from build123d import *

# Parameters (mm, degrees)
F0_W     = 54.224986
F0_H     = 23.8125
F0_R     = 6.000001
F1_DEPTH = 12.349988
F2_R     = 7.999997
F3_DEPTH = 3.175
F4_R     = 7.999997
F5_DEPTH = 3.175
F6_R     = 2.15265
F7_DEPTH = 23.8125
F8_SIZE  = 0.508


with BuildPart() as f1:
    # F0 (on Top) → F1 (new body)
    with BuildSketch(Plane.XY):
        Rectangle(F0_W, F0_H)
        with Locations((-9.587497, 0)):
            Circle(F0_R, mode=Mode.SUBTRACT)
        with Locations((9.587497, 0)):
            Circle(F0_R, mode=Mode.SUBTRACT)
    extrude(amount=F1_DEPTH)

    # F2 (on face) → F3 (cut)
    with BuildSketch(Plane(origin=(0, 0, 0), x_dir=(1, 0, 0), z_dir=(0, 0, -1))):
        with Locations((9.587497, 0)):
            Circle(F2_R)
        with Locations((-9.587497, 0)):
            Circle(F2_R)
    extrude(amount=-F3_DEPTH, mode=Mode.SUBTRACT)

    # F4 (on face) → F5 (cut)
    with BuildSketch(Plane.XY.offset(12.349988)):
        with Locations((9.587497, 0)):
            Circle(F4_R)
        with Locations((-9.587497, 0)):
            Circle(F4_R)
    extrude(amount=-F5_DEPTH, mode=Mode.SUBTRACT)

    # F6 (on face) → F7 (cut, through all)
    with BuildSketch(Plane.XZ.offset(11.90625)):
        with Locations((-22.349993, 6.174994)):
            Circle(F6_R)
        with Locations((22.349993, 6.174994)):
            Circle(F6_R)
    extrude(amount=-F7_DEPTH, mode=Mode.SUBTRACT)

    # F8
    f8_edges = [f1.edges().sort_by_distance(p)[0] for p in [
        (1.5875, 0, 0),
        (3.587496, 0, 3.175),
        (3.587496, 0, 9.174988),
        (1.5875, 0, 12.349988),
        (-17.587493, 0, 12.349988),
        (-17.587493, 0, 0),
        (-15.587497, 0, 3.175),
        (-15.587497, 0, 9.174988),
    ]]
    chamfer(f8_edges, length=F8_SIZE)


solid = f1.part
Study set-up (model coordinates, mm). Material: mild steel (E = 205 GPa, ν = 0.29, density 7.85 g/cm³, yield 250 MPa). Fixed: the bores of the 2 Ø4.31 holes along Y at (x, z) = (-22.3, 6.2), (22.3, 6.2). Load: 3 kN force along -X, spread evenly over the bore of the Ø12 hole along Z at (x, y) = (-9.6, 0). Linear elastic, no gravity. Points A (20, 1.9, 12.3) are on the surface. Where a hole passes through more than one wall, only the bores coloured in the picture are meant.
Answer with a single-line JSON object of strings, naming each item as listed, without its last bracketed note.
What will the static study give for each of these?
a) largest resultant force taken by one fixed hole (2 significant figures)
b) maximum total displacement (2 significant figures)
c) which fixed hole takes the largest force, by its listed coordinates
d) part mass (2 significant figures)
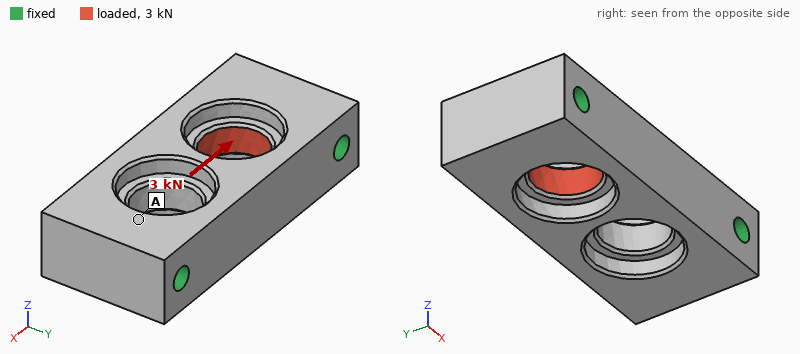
{"largest resultant force taken by one fixed hole": "2.2 kN", "maximum total displacement": "1.5 µm", "which fixed hole takes the largest force, by its listed coordinates": "(-22.3, 6.2)", "part mass": "89 g"}
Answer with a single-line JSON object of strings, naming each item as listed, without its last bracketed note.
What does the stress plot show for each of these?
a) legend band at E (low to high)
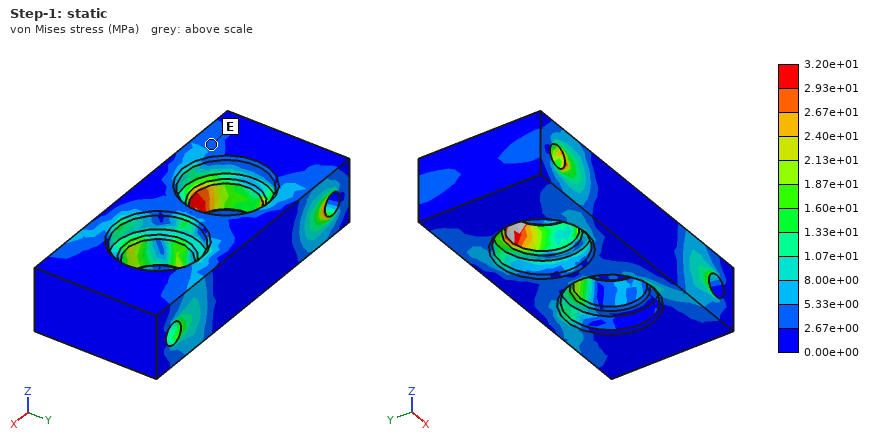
{"legend band at E": "2.67e+00 to 5.33e+00 MPa"}
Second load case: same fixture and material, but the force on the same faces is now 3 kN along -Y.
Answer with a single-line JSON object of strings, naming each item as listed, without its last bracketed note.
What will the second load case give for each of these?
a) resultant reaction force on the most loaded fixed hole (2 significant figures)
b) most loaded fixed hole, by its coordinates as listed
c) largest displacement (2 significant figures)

{"resultant reaction force on the most loaded fixed hole": "2.3 kN", "most loaded fixed hole, by its coordinates as listed": "(-22.3, 6.2)", "largest displacement": "4.1 µm"}
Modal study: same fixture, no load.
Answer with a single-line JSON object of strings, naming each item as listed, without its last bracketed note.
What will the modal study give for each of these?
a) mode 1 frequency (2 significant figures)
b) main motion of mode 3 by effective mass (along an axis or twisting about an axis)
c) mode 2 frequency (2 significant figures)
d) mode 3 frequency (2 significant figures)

{"mode 1 frequency": "20 kHz", "main motion of mode 3 by effective mass": "twisting about X", "mode 2 frequency": "21 kHz", "mode 3 frequency": "25 kHz"}
